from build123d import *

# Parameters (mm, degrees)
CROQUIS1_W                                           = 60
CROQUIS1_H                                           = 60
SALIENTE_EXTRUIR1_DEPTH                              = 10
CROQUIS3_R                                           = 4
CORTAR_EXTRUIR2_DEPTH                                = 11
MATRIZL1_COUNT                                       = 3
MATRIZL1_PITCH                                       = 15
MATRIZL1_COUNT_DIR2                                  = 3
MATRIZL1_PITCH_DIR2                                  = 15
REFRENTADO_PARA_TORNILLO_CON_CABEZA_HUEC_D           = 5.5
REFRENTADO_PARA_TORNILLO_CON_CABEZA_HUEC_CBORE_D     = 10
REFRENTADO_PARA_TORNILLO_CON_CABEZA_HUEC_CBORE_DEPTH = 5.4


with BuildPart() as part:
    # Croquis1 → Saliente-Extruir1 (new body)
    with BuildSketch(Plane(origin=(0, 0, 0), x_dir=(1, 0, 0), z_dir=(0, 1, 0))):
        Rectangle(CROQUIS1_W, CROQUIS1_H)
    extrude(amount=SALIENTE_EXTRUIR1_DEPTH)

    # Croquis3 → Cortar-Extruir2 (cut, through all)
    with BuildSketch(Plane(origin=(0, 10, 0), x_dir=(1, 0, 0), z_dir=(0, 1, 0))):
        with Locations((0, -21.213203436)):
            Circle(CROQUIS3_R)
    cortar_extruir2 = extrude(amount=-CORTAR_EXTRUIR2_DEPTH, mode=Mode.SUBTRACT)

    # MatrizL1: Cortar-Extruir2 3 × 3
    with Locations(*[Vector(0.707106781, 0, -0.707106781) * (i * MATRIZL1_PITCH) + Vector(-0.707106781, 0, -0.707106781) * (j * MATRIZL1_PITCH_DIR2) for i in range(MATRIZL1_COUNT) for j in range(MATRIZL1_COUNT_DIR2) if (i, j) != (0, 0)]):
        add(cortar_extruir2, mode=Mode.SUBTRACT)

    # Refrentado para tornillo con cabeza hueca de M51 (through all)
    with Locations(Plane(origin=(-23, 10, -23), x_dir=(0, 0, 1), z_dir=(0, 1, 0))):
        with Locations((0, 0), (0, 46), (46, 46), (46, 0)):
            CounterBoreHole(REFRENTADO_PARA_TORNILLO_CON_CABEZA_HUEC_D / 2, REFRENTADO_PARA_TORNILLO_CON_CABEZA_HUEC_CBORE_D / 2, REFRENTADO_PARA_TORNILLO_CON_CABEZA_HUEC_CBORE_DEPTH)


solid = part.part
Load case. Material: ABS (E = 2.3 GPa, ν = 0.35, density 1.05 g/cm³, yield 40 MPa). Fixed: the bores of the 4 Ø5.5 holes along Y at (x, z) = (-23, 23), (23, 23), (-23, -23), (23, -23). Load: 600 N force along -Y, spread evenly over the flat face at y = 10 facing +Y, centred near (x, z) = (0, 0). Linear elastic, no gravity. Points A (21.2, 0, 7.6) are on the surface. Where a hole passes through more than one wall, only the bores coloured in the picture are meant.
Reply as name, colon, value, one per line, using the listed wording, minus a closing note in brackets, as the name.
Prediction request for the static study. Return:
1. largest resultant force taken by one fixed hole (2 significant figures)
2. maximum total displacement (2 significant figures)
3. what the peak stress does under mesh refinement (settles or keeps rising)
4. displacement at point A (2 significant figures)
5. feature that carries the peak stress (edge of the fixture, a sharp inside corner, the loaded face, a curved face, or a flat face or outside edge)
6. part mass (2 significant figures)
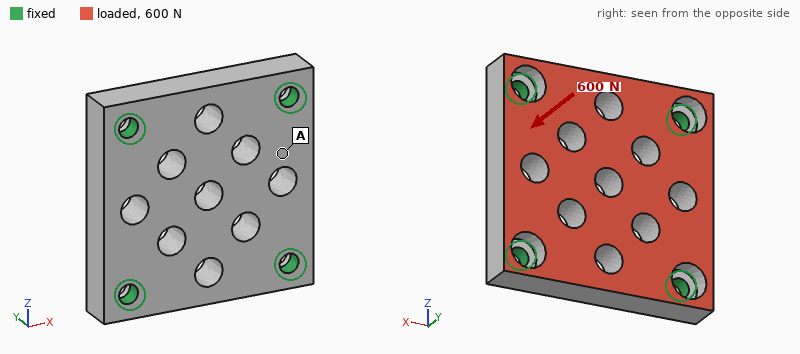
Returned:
largest resultant force taken by one fixed hole: 180 N
maximum total displacement: 66 µm
what the peak stress does under mesh refinement: keeps rising
displacement at point A: 38 µm
feature that carries the peak stress: edge of the fixture
part mass: 31 g
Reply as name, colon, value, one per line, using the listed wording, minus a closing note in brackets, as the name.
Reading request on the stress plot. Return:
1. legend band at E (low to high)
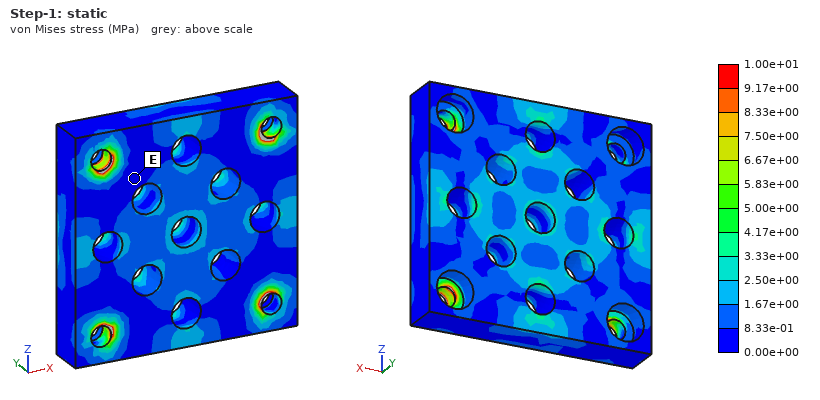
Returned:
legend band at E: 0.00e+00 to 8.33e-01 MPa
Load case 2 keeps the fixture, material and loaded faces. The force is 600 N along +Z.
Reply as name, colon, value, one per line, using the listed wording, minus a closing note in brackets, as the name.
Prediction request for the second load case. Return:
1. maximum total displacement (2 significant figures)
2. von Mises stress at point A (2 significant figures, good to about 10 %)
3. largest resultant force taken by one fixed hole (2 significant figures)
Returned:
maximum total displacement: 28 µm
von Mises stress at point A: 0.63 MPa
largest resultant force taken by one fixed hole: 160 N
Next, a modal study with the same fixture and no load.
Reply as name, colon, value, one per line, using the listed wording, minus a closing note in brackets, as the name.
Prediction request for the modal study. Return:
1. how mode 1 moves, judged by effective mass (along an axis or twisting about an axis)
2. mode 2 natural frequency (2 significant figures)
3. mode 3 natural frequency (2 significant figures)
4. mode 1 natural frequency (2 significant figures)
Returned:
how mode 1 moves, judged by effective mass: along Y
mode 2 natural frequency: 4900 Hz
mode 3 natural frequency: 5000 Hz
mode 1 natural frequency: 3300 Hz
